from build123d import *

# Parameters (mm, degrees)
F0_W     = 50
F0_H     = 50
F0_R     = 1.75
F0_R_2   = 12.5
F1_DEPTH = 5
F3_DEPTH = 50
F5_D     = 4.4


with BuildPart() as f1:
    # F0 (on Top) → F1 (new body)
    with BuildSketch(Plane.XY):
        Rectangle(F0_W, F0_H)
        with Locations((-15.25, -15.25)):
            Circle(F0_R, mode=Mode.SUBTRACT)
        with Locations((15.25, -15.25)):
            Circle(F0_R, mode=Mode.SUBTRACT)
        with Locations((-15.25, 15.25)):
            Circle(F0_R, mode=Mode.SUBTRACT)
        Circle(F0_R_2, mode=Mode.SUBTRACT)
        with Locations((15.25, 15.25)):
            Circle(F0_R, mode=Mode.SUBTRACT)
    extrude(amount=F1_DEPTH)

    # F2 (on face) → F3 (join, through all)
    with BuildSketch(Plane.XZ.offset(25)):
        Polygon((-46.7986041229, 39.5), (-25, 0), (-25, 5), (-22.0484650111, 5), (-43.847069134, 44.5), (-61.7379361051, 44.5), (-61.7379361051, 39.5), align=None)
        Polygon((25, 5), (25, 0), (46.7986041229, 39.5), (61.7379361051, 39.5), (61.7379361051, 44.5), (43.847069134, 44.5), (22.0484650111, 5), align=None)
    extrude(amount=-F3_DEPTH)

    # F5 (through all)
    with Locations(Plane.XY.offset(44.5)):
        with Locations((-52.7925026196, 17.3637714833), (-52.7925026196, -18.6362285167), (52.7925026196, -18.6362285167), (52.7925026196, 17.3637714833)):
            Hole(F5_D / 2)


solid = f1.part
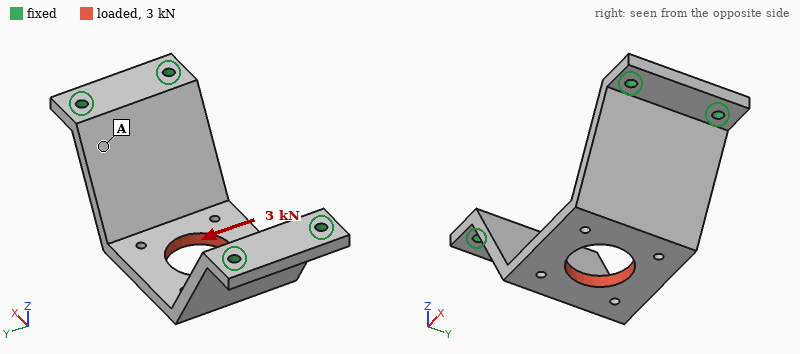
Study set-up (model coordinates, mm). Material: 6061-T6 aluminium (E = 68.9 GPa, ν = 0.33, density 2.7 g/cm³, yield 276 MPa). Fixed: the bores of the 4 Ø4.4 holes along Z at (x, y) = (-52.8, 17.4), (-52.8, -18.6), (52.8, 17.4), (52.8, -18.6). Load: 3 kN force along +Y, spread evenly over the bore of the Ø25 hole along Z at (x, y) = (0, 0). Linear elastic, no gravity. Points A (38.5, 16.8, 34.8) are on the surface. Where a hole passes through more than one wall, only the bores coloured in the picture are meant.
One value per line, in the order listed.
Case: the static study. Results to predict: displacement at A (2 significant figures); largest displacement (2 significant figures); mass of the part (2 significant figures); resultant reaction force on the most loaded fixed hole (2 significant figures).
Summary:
25 µm
77 µm
110 g
2.1 kN
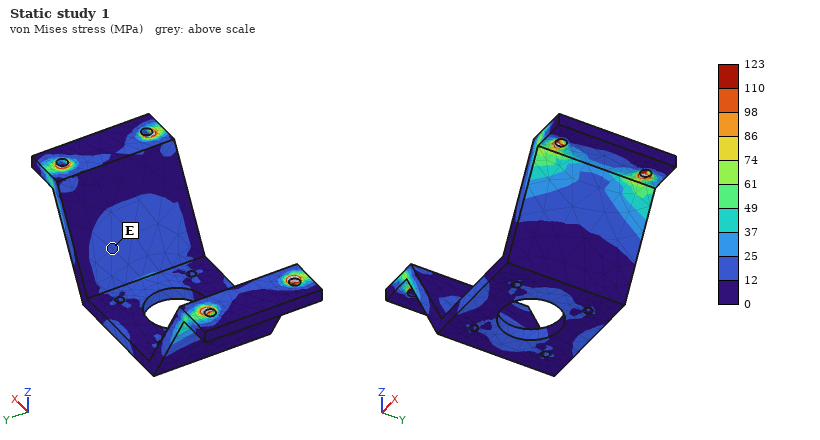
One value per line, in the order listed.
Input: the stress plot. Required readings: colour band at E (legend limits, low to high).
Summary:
12 to 25 MPa
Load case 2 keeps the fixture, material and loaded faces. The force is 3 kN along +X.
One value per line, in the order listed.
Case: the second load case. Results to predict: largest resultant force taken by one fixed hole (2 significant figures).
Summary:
930 N
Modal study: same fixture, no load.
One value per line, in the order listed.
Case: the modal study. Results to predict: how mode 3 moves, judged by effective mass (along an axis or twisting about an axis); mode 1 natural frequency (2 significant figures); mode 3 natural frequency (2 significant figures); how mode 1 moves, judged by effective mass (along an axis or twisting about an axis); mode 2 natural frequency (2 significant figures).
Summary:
along Y
2300 Hz
4700 Hz
along X
4400 Hz
